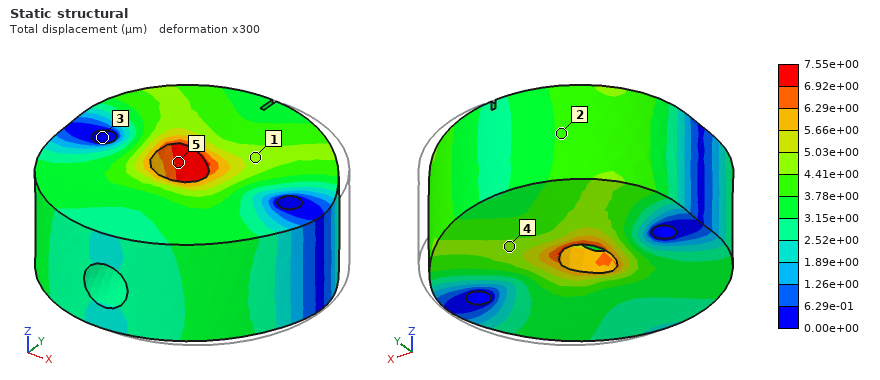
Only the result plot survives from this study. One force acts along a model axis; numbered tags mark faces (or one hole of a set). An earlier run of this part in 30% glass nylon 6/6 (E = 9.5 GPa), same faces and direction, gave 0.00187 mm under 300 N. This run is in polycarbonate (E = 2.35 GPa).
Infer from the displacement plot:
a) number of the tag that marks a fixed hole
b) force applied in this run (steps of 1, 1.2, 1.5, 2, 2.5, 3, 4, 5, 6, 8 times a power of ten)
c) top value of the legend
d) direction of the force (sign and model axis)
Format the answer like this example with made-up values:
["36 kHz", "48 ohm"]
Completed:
["3", "300 N", "7.55e+00 µm", "-X"]
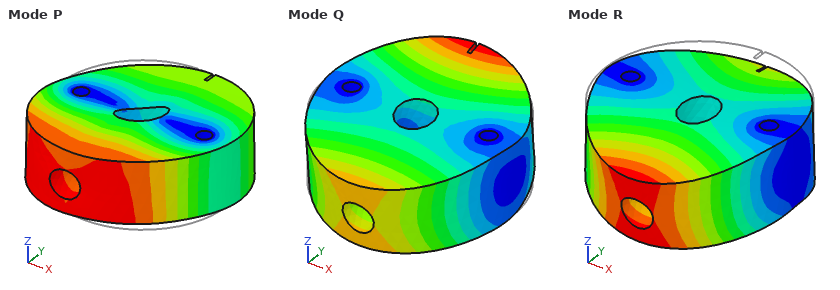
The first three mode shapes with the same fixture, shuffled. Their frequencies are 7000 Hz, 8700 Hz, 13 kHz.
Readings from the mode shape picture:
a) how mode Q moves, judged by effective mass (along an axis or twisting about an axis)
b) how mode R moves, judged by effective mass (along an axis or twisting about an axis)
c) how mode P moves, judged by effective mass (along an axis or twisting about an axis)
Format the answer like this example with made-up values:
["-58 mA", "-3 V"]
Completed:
["twisting about X", "along Z", "twisting about Z"]
